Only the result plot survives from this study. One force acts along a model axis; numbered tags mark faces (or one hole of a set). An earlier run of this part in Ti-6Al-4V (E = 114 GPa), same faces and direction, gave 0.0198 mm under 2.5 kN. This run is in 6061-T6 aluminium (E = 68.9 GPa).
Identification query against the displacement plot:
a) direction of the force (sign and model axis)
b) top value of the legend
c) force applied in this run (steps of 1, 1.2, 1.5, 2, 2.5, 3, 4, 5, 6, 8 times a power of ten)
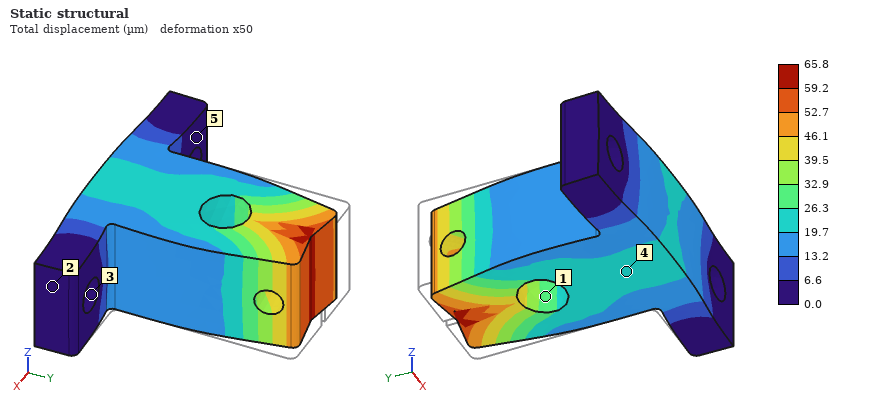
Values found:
-Y
65.8 µm
5 kN
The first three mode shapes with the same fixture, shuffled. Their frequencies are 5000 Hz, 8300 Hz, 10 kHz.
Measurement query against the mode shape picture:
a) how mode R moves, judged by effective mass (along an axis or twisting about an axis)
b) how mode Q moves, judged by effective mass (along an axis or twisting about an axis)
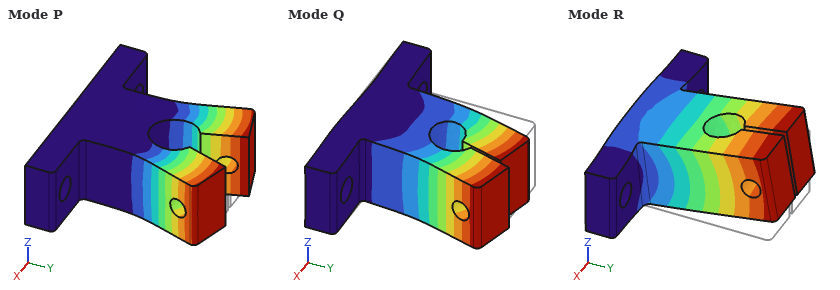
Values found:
along Z
along X
